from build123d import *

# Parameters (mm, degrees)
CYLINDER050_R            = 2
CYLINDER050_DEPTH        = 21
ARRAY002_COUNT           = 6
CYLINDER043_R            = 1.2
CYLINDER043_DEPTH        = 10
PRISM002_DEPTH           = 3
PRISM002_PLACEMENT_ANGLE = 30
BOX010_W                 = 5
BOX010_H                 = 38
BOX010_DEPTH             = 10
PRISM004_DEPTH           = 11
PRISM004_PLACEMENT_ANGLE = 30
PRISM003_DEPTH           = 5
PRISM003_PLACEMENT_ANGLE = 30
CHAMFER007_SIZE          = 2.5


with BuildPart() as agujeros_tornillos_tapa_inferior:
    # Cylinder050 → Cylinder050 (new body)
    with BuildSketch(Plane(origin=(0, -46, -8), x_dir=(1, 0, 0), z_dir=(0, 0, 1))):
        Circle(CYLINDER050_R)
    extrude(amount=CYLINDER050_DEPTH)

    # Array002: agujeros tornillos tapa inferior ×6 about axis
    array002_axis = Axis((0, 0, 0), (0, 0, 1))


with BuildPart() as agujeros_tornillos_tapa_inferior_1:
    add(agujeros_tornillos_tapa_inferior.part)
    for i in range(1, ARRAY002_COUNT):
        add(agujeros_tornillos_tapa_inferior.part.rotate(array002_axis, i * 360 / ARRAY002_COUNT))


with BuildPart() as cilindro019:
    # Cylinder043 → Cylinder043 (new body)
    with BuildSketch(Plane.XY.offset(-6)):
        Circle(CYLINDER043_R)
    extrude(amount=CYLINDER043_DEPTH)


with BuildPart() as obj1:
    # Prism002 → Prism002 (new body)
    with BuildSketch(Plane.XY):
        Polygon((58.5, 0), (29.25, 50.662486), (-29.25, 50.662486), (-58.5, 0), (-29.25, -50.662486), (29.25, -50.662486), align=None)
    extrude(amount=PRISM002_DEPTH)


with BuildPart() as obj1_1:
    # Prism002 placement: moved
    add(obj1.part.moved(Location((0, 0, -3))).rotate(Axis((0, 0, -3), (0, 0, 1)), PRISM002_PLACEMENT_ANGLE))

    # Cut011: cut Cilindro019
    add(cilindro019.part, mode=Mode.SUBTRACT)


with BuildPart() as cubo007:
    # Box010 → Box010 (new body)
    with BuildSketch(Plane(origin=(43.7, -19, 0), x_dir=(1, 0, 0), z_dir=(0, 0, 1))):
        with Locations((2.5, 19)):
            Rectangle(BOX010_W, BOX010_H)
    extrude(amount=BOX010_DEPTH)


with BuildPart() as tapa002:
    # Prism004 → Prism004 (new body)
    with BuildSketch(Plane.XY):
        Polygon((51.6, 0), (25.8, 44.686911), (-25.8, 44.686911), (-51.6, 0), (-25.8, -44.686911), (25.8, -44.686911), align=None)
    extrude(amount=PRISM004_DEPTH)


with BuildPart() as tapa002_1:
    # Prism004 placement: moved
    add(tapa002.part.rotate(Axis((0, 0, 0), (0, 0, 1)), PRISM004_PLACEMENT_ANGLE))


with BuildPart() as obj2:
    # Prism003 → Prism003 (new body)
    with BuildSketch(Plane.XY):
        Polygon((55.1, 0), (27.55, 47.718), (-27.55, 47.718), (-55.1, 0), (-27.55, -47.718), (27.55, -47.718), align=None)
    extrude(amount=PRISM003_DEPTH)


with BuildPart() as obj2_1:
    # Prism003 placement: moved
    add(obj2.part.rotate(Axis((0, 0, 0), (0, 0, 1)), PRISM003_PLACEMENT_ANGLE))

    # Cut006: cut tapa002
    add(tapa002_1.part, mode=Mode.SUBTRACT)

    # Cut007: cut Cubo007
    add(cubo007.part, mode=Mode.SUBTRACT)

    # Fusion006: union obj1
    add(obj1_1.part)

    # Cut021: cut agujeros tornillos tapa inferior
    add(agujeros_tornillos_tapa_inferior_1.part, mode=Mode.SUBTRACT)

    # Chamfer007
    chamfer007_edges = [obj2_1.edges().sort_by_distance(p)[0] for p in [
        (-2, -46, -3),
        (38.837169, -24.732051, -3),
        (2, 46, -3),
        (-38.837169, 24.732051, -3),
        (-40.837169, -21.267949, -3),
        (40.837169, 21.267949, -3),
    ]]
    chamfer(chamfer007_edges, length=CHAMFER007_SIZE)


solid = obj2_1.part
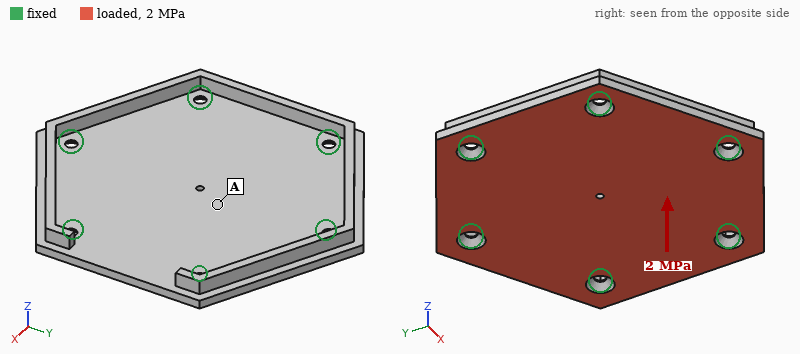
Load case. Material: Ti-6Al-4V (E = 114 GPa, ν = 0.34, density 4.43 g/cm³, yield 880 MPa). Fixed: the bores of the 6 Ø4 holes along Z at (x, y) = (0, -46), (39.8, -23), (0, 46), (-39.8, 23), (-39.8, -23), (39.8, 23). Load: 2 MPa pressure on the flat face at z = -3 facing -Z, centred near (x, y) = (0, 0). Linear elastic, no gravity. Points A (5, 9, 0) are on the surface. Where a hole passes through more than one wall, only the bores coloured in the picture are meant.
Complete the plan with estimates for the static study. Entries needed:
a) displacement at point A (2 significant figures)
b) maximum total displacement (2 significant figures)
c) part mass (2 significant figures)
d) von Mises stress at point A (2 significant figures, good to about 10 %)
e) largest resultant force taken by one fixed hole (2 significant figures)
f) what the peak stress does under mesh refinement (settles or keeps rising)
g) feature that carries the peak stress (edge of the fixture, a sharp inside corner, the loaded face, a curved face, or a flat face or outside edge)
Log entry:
0.81 mm
0.88 mm
130 g
270 MPa
5.9 kN
keeps rising
edge of the fixture
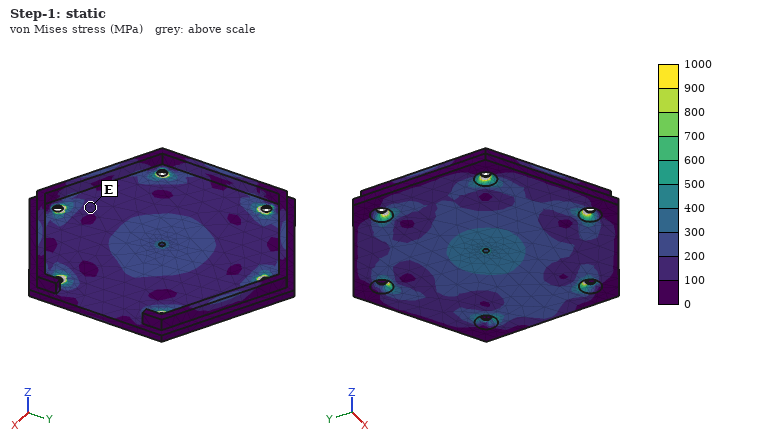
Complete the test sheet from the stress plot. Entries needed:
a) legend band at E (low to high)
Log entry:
100 to 200 MPa
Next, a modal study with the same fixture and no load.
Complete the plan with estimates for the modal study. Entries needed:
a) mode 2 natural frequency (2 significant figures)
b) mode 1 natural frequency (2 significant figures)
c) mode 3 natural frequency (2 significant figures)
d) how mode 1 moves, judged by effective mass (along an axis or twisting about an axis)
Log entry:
5200 Hz
2600 Hz
5400 Hz
along Z
